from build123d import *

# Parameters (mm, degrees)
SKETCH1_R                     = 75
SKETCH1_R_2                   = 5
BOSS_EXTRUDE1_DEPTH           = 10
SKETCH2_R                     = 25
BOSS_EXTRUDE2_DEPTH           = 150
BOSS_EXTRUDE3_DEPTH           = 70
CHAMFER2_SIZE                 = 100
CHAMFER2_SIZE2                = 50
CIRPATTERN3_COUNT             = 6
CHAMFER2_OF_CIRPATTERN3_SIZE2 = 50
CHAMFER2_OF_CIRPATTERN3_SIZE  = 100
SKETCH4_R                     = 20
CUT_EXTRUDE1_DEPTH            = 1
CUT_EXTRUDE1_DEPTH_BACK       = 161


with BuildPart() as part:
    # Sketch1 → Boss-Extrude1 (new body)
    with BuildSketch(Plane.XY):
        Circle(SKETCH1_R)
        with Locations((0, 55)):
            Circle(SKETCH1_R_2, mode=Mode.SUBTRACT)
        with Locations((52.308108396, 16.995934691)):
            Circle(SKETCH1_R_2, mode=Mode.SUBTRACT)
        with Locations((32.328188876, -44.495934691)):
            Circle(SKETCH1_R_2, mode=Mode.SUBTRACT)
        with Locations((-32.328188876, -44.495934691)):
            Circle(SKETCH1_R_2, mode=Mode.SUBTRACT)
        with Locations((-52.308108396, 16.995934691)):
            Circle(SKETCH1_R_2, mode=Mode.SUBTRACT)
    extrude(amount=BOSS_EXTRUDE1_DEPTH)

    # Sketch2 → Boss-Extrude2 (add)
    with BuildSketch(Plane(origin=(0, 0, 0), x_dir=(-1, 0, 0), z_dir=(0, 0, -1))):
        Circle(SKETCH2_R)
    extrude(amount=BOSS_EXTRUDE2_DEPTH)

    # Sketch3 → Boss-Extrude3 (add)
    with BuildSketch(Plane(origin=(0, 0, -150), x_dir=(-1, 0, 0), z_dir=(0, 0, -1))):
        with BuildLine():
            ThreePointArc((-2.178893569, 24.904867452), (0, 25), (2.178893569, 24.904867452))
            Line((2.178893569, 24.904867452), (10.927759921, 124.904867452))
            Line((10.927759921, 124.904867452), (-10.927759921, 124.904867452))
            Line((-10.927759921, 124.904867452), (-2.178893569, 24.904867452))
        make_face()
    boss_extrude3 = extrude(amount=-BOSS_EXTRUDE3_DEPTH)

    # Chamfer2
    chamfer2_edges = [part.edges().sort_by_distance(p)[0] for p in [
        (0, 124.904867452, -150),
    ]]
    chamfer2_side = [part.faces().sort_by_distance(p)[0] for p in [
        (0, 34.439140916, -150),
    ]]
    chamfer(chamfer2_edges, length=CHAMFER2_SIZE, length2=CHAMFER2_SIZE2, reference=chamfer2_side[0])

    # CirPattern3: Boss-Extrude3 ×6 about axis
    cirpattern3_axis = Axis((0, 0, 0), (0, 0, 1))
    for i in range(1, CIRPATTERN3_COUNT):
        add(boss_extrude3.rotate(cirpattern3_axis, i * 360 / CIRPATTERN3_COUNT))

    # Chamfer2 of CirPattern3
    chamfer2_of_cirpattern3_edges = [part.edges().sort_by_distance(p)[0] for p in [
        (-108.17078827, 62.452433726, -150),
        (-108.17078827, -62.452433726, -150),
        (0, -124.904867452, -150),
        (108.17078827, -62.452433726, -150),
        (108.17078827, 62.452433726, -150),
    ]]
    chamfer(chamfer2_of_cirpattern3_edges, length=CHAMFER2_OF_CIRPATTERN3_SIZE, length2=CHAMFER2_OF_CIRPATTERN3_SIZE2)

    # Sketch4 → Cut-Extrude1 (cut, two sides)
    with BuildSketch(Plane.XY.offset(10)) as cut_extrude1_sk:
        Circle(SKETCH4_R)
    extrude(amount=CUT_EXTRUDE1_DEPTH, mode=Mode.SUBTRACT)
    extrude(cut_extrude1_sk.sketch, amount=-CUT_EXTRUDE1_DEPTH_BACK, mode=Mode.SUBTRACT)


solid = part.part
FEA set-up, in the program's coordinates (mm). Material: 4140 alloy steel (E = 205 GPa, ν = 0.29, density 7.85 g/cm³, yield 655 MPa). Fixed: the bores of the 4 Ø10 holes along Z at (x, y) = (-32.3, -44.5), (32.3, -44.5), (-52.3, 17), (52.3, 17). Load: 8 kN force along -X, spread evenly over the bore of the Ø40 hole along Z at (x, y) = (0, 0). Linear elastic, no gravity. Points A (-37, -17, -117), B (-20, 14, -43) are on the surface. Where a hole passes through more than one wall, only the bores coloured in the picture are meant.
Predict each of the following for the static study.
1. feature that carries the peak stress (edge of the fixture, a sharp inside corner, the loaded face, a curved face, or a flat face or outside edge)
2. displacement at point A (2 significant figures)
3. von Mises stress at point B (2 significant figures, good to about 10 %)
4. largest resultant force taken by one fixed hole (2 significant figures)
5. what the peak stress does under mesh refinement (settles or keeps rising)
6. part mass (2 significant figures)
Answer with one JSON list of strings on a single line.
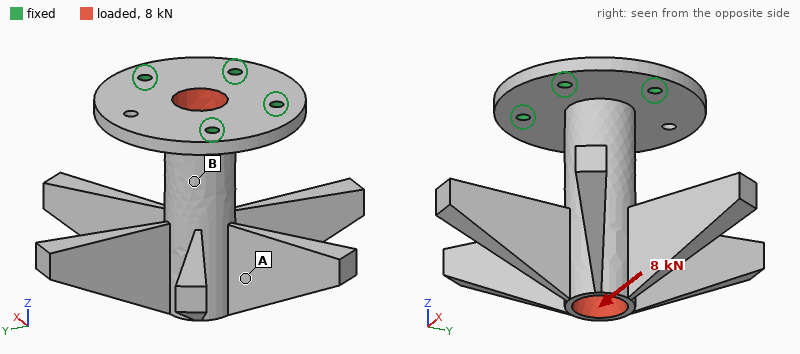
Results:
["edge of the fixture", "0.24 mm", "36 MPa", "6.2 kN", "keeps rising", "4.5 kg"]
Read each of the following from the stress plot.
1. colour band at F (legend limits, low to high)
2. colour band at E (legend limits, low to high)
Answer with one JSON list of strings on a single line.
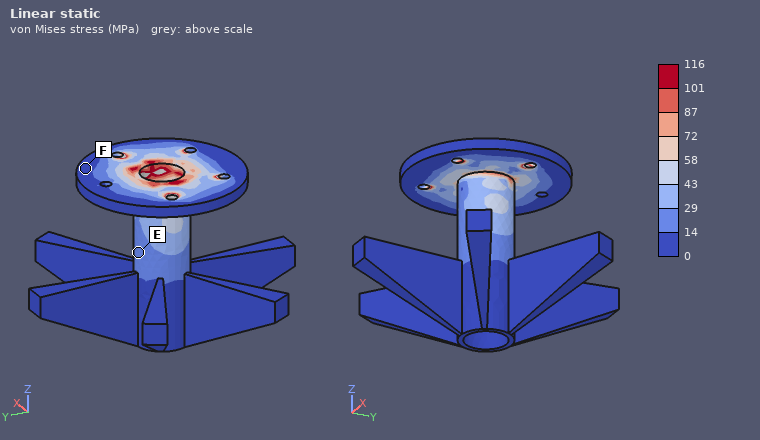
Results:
["0 to 14 MPa", "14 to 29 MPa"]
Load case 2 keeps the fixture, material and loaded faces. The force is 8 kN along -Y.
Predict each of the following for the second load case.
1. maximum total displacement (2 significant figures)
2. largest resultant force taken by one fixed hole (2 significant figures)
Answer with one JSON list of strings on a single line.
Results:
["0.42 mm", "5.7 kN"]
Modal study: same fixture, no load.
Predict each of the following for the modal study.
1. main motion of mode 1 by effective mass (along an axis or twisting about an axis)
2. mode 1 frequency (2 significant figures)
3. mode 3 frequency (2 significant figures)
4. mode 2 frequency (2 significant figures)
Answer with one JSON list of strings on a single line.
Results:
["along Y", "320 Hz", "360 Hz", "350 Hz"]
